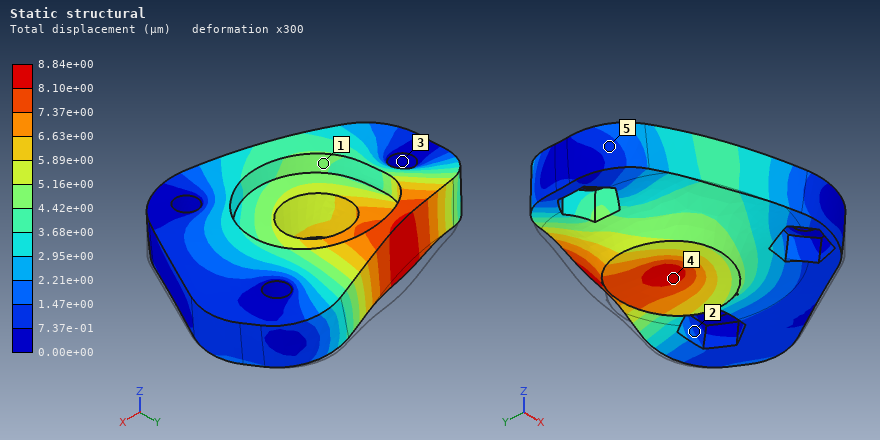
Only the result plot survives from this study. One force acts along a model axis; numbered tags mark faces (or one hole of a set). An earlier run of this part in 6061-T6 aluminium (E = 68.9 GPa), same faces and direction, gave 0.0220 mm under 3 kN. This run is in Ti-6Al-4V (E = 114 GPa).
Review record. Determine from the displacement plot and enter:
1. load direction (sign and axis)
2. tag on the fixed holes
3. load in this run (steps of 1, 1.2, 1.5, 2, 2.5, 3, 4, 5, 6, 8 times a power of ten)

+Z
3
2 kN
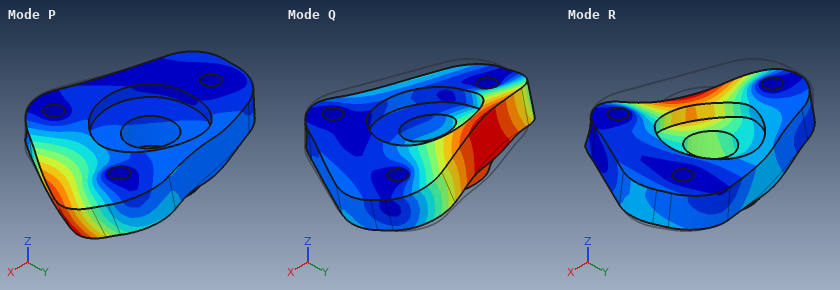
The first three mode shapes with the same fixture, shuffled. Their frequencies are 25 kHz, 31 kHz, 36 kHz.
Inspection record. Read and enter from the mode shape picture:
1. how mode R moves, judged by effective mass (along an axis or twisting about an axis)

along Z
